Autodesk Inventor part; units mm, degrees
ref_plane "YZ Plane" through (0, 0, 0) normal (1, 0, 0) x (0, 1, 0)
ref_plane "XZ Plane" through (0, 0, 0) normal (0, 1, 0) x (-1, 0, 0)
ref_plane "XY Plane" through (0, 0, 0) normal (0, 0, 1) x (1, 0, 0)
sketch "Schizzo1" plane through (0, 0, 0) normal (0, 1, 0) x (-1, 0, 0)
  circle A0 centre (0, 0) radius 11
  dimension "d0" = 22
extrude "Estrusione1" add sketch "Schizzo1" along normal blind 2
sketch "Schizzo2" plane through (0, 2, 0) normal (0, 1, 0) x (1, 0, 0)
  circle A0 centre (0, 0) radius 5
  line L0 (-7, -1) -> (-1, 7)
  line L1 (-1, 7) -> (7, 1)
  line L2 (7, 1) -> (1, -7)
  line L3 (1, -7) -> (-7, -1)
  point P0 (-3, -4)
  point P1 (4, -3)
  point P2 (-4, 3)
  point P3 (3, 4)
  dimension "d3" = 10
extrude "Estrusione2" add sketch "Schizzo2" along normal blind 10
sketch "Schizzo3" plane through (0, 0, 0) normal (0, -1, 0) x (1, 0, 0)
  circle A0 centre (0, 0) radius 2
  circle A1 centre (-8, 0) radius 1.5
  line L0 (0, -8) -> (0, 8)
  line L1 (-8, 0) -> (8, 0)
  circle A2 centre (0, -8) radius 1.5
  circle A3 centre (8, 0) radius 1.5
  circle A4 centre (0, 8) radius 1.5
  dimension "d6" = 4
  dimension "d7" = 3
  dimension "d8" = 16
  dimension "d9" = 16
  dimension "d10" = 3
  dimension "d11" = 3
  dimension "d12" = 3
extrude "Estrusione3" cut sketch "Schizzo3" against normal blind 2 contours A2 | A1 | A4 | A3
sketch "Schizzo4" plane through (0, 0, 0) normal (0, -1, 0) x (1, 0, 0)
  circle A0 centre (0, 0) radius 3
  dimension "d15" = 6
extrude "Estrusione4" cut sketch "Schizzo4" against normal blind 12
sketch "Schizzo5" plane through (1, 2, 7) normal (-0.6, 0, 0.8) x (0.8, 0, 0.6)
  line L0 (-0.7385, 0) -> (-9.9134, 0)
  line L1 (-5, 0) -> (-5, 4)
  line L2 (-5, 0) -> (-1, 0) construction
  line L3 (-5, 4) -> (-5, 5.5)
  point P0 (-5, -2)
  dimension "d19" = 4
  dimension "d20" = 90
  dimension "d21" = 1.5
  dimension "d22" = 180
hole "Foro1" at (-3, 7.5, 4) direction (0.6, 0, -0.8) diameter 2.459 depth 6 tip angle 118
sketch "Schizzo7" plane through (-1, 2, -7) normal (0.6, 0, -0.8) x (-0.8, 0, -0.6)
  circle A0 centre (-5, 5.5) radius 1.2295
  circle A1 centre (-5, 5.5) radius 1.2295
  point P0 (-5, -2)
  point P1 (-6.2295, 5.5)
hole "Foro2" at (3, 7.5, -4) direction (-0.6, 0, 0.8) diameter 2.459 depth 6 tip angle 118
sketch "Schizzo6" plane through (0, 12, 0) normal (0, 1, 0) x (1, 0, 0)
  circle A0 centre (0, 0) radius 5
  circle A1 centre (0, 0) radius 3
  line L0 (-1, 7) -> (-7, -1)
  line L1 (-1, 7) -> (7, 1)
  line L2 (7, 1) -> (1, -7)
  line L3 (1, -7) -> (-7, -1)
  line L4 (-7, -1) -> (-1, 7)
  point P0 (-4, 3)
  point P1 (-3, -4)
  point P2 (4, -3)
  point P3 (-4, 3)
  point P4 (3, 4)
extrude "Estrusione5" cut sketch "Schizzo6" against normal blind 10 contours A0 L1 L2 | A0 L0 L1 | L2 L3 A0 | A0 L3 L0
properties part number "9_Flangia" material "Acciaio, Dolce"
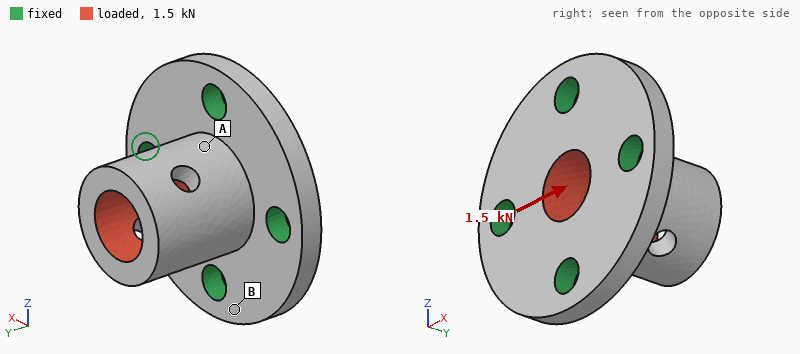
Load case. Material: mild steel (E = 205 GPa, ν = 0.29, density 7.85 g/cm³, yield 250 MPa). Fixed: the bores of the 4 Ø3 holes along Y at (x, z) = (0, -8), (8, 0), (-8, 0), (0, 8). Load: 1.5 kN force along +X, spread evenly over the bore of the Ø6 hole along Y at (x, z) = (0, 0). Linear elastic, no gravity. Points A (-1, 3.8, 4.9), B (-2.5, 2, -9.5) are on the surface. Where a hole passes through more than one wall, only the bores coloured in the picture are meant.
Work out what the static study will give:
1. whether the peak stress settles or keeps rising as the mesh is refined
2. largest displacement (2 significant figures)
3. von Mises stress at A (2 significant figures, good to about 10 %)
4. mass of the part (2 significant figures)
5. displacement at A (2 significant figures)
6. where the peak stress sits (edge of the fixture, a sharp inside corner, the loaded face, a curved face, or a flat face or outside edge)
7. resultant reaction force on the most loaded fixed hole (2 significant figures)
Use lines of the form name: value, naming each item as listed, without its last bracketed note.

whether the peak stress settles or keeps rising as the mesh is refined: keeps rising
largest displacement: 12 µm
von Mises stress at A: 37 MPa
mass of the part: 8.9 g
displacement at A: 2.7 µm
where the peak stress sits: edge of the fixture
resultant reaction force on the most loaded fixed hole: 750 N
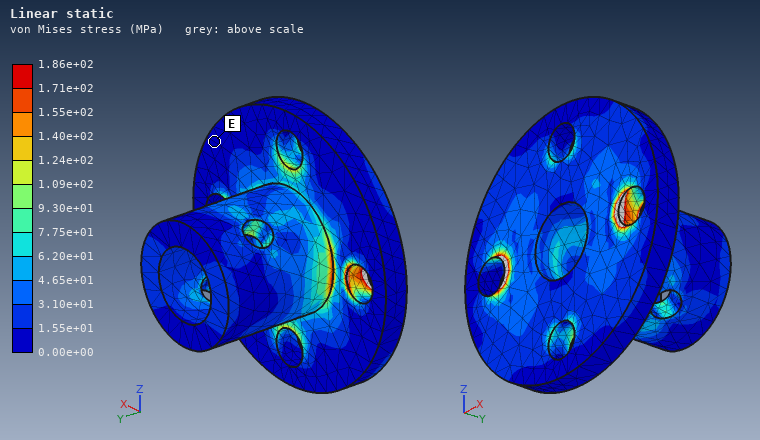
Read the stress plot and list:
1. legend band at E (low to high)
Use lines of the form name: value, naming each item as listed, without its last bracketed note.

legend band at E: 0.00e+00 to 1.55e+01 MPa
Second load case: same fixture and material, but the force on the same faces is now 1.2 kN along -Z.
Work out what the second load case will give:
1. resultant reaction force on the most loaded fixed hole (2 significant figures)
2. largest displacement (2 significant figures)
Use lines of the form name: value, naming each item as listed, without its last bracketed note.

resultant reaction force on the most loaded fixed hole: 600 N
largest displacement: 9.4 µm
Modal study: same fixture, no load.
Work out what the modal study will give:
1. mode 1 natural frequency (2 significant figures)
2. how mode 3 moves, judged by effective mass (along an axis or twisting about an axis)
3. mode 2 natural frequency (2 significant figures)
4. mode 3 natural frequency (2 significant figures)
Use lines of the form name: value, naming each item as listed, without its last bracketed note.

mode 1 natural frequency: 30 kHz
how mode 3 moves, judged by effective mass: along Y
mode 2 natural frequency: 31 kHz
mode 3 natural frequency: 54 kHz
